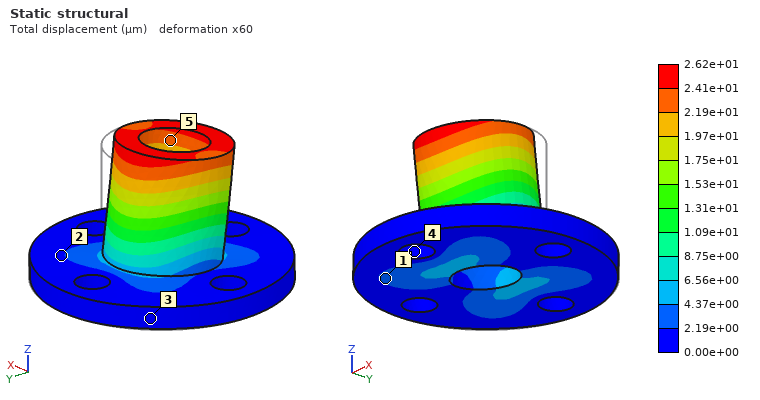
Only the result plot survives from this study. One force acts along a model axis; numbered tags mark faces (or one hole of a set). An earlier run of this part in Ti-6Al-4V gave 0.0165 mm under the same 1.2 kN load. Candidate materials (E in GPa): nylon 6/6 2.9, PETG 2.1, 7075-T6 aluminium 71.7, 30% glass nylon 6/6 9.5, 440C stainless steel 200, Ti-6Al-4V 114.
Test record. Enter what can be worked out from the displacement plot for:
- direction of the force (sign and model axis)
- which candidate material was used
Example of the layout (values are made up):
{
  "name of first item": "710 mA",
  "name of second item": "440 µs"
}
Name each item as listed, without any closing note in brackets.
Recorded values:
{
  "direction of the force": "-Y",
  "which candidate material was used": "7075-T6 aluminium"
}
